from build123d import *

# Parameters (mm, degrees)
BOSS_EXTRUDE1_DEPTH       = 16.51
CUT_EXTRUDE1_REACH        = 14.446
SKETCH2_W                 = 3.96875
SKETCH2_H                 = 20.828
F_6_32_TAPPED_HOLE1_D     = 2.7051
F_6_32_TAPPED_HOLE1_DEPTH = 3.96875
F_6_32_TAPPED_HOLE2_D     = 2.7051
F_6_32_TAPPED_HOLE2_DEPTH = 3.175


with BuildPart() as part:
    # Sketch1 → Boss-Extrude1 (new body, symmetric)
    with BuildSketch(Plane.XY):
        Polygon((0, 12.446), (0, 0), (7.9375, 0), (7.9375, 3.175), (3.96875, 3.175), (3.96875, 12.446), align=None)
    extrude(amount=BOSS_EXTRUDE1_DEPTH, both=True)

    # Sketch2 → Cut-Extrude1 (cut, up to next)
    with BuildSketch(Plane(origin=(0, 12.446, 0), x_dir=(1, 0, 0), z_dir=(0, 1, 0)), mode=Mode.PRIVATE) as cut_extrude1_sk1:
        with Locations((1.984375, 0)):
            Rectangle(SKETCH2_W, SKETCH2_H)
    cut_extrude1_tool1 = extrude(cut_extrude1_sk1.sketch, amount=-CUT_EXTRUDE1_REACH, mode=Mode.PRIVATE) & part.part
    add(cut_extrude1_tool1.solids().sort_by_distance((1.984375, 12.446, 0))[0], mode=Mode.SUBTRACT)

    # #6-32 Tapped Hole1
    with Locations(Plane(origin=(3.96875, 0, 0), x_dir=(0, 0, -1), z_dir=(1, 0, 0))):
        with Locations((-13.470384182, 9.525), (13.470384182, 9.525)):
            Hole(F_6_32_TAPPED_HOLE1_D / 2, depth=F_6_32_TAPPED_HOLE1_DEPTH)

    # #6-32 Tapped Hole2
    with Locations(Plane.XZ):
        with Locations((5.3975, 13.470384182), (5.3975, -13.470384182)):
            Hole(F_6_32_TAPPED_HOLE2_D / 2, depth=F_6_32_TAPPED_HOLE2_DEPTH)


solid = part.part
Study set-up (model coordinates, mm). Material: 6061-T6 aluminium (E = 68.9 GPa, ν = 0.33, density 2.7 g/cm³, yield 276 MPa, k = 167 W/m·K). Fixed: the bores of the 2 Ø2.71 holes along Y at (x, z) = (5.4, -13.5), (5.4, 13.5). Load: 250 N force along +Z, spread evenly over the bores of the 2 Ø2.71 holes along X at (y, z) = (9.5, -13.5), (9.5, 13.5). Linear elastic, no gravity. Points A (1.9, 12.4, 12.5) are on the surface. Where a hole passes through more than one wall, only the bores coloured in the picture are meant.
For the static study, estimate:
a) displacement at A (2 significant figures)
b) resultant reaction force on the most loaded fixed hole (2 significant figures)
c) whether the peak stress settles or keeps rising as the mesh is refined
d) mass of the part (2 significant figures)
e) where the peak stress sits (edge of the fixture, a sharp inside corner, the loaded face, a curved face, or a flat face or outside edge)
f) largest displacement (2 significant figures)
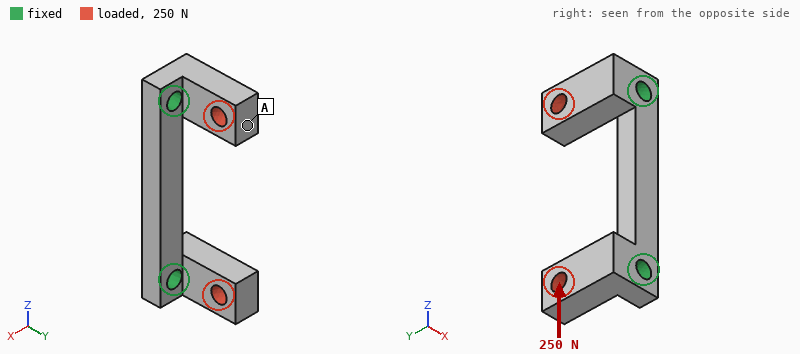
20 µm
130 N
keeps rising
2.5 g
edge of the fixture
20 µm
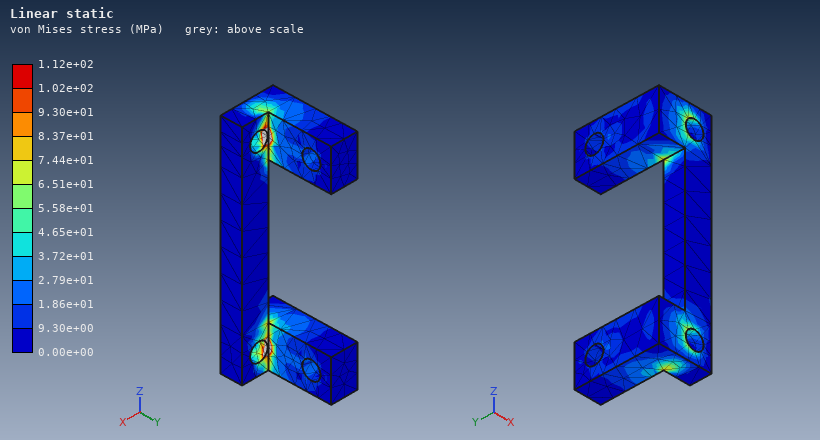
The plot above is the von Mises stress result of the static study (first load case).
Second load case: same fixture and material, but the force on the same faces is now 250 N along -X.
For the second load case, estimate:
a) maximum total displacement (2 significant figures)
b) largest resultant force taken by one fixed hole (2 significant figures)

33 µm
130 N
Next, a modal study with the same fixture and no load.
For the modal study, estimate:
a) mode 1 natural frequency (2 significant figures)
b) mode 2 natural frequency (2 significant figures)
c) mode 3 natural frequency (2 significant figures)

19 kHz
19 kHz
22 kHz
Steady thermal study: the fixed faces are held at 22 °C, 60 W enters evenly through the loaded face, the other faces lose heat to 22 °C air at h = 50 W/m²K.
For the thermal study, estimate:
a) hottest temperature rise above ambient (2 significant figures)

81 K
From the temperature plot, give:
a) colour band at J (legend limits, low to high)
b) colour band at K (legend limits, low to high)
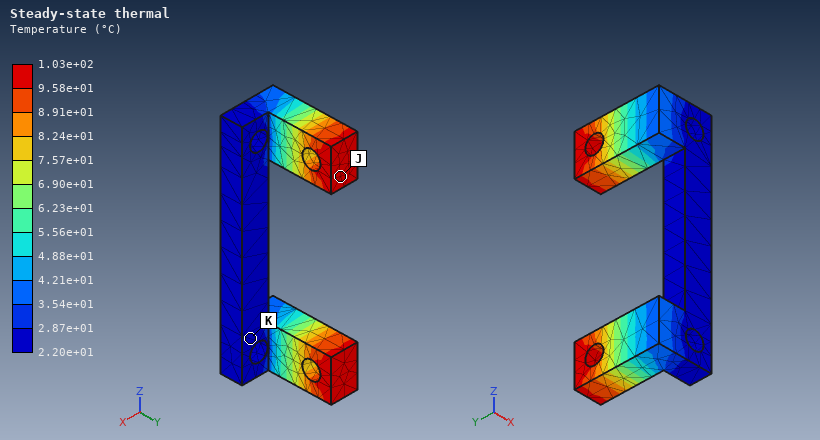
9.58e+01 to 1.03e+02 °C
2.20e+01 to 2.87e+01 °C
